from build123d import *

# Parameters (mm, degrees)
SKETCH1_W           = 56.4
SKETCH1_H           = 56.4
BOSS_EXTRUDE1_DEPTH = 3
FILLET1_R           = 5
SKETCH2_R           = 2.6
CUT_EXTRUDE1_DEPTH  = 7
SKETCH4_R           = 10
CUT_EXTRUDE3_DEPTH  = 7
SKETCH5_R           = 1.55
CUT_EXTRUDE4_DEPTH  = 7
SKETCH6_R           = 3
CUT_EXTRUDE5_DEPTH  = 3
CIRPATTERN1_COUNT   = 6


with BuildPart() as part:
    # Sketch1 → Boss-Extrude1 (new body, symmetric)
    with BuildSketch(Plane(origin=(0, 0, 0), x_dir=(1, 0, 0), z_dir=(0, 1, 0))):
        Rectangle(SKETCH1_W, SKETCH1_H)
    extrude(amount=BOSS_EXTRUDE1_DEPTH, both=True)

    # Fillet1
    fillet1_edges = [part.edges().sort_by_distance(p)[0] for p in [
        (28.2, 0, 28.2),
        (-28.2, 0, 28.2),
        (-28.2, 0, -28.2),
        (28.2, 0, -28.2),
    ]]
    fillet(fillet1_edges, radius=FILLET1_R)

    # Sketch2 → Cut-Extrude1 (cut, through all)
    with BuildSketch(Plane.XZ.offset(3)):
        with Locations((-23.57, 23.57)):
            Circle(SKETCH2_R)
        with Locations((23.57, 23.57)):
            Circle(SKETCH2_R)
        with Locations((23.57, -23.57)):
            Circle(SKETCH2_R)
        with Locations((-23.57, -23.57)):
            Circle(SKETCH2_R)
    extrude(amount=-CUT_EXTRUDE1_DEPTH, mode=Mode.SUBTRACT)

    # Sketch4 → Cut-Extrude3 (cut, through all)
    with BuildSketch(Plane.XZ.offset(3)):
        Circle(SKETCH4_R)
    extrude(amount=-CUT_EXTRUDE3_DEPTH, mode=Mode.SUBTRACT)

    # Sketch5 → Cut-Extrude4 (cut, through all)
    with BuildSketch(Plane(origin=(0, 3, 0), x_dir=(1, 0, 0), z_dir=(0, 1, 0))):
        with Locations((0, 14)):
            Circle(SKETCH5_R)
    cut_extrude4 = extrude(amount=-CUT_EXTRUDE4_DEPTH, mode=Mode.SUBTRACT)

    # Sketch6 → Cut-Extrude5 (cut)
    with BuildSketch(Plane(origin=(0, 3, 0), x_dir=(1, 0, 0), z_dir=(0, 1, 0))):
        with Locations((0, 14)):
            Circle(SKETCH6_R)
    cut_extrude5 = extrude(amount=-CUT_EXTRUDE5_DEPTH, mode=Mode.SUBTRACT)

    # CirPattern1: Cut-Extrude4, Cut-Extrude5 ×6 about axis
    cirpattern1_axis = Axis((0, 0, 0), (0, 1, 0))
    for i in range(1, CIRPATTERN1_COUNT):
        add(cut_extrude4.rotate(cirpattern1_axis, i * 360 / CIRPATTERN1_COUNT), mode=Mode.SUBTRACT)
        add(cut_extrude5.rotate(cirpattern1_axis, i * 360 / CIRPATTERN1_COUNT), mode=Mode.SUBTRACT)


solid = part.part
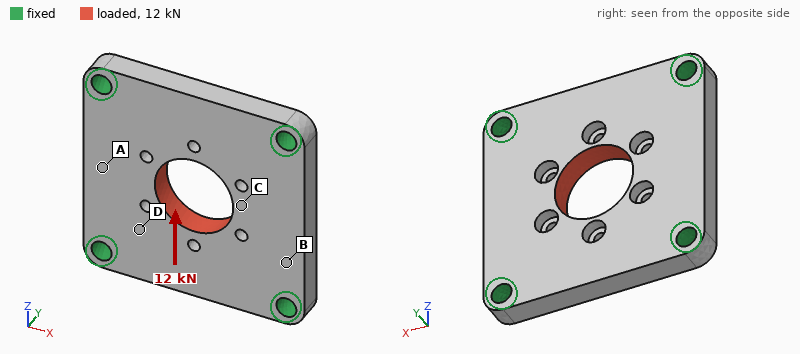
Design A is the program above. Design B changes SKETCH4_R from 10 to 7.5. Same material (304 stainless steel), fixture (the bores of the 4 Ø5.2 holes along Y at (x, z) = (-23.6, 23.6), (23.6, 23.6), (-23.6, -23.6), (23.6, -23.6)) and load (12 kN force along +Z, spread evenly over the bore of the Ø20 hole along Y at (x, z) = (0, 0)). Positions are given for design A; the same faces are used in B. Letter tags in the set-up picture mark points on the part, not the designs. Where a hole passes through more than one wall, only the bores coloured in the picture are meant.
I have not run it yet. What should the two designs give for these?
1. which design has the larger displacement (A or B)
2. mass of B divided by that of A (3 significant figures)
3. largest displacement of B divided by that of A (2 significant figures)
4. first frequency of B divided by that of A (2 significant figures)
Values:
A
1.05
0.83
0.95
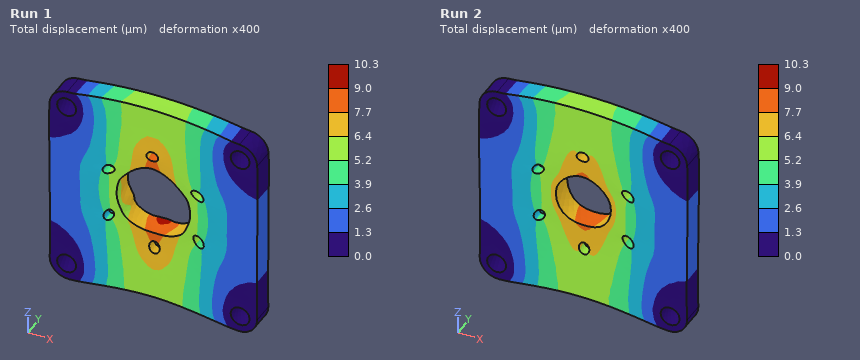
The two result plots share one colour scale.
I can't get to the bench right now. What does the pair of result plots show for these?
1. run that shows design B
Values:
Run 2
